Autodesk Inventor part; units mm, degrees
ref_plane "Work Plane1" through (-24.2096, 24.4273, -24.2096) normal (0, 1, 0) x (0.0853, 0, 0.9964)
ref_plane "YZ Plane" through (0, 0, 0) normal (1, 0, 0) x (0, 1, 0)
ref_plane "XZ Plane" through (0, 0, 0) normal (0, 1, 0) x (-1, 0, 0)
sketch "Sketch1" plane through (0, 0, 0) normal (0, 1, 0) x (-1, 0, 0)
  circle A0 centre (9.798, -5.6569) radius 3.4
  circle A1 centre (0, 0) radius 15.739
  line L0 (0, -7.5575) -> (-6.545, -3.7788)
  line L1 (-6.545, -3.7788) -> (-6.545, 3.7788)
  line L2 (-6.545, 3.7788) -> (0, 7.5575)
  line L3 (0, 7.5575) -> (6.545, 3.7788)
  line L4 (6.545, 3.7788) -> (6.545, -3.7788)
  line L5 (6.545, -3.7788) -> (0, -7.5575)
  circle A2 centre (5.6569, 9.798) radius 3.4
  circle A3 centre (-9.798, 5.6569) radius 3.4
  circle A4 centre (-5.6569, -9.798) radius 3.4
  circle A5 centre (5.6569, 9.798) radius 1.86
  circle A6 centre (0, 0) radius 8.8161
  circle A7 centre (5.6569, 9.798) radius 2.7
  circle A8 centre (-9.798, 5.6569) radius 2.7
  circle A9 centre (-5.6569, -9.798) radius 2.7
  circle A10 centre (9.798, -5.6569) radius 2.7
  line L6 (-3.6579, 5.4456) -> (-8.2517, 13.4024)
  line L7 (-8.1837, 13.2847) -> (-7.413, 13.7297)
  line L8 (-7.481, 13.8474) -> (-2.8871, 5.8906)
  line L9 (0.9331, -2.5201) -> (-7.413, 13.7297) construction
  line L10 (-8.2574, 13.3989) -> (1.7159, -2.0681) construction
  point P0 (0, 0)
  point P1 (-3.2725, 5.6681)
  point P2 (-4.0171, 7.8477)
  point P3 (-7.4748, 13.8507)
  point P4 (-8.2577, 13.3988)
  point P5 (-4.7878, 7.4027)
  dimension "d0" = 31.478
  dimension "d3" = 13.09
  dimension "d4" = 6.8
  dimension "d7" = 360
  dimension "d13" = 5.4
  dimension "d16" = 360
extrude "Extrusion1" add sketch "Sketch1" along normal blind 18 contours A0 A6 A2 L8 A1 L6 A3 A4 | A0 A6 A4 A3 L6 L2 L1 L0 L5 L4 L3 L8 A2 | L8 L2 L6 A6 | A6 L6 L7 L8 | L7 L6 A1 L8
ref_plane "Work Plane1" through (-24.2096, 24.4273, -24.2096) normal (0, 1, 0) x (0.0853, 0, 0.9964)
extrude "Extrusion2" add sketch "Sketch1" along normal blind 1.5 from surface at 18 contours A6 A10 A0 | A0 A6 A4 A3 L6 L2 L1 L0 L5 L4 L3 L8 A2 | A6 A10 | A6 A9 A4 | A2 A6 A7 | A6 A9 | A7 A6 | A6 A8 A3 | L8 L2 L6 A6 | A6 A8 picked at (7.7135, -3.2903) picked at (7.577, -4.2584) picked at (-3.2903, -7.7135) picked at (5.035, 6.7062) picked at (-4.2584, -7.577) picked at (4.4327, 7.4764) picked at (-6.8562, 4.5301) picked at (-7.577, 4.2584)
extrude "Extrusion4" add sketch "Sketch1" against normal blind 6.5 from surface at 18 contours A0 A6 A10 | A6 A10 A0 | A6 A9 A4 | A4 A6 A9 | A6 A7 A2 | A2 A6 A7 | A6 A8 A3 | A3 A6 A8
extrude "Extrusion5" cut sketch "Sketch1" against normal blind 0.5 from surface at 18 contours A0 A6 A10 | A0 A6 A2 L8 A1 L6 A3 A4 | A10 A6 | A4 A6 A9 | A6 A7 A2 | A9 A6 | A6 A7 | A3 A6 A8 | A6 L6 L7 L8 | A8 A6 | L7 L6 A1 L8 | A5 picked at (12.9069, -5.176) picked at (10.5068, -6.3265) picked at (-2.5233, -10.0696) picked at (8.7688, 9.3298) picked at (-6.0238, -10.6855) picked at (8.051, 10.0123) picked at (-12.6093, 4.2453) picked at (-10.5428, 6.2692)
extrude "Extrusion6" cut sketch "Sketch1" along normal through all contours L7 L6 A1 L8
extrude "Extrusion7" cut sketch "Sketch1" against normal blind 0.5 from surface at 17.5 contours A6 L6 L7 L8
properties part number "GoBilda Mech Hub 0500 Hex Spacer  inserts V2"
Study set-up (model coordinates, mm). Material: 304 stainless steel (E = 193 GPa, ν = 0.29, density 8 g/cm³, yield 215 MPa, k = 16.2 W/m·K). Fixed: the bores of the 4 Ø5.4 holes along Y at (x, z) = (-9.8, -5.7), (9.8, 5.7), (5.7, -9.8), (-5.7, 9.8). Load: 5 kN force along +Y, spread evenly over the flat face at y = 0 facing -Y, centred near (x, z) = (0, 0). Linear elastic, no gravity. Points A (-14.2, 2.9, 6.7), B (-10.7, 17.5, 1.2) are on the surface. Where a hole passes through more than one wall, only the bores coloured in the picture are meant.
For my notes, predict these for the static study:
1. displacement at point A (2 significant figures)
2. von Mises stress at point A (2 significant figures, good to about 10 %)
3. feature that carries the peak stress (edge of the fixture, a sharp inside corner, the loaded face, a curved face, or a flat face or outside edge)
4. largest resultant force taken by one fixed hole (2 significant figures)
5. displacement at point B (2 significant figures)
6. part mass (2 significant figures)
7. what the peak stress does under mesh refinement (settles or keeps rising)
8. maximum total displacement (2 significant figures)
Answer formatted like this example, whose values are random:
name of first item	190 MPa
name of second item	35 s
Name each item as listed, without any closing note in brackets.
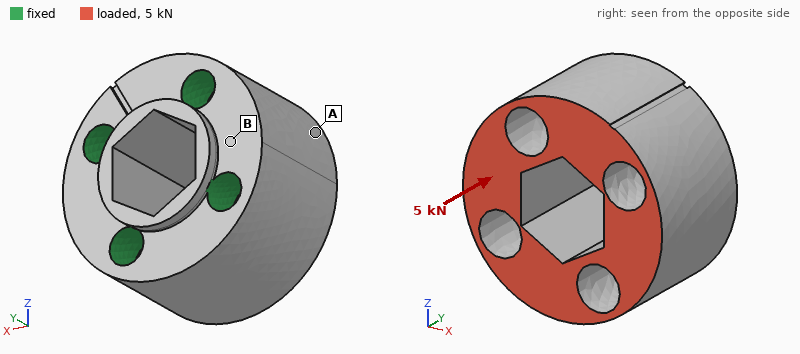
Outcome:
displacement at point A	1.1 µm
von Mises stress at point A	9.9 MPa
feature that carries the peak stress	edge of the fixture
largest resultant force taken by one fixed hole	1.3 kN
displacement at point B	0.45 µm
part mass	72 g
what the peak stress does under mesh refinement	keeps rising
maximum total displacement	1.3 µm
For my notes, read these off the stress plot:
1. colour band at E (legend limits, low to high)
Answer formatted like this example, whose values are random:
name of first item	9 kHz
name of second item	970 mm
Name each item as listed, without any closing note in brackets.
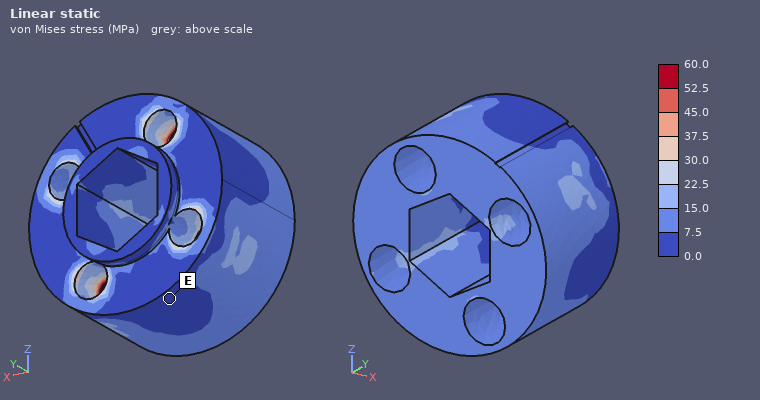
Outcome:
colour band at E	0.0 to 7.5 MPa
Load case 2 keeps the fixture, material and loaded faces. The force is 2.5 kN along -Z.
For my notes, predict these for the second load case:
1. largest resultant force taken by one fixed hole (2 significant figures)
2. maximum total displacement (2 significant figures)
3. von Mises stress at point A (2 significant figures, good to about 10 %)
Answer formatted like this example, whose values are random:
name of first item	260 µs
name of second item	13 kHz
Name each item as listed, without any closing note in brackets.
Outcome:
largest resultant force taken by one fixed hole	1.2 kN
maximum total displacement	4.2 µm
von Mises stress at point A	9.5 MPa
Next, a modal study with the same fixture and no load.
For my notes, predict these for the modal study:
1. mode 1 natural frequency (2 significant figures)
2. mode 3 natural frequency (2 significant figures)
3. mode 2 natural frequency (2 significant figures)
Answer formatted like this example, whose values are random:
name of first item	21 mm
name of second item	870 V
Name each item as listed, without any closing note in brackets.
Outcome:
mode 1 natural frequency	29 kHz
mode 3 natural frequency	32 kHz
mode 2 natural frequency	31 kHz
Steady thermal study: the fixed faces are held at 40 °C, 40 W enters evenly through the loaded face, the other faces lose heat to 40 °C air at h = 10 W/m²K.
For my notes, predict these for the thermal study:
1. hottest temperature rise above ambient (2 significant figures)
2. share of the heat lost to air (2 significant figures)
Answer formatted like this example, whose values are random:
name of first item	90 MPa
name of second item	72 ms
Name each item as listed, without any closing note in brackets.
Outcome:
hottest temperature rise above ambient	78 K
share of the heat lost to air	3.5 %
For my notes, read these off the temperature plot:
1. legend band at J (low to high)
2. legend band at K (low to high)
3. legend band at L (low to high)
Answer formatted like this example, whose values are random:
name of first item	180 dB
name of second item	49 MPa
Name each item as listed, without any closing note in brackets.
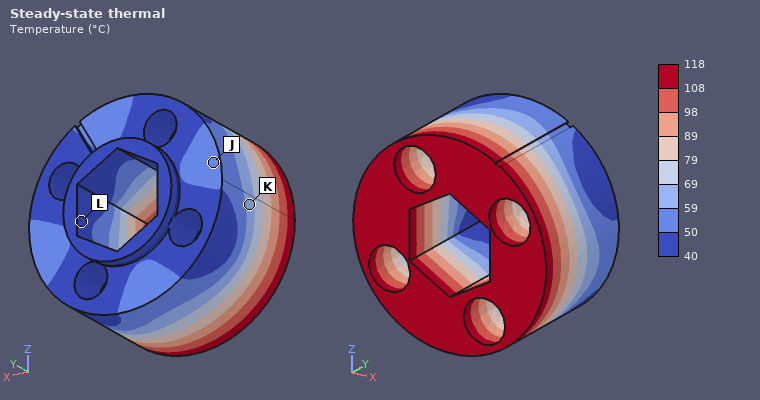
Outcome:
legend band at J	50 to 59 °C
legend band at K	59 to 69 °C
legend band at L	40 to 50 °C
